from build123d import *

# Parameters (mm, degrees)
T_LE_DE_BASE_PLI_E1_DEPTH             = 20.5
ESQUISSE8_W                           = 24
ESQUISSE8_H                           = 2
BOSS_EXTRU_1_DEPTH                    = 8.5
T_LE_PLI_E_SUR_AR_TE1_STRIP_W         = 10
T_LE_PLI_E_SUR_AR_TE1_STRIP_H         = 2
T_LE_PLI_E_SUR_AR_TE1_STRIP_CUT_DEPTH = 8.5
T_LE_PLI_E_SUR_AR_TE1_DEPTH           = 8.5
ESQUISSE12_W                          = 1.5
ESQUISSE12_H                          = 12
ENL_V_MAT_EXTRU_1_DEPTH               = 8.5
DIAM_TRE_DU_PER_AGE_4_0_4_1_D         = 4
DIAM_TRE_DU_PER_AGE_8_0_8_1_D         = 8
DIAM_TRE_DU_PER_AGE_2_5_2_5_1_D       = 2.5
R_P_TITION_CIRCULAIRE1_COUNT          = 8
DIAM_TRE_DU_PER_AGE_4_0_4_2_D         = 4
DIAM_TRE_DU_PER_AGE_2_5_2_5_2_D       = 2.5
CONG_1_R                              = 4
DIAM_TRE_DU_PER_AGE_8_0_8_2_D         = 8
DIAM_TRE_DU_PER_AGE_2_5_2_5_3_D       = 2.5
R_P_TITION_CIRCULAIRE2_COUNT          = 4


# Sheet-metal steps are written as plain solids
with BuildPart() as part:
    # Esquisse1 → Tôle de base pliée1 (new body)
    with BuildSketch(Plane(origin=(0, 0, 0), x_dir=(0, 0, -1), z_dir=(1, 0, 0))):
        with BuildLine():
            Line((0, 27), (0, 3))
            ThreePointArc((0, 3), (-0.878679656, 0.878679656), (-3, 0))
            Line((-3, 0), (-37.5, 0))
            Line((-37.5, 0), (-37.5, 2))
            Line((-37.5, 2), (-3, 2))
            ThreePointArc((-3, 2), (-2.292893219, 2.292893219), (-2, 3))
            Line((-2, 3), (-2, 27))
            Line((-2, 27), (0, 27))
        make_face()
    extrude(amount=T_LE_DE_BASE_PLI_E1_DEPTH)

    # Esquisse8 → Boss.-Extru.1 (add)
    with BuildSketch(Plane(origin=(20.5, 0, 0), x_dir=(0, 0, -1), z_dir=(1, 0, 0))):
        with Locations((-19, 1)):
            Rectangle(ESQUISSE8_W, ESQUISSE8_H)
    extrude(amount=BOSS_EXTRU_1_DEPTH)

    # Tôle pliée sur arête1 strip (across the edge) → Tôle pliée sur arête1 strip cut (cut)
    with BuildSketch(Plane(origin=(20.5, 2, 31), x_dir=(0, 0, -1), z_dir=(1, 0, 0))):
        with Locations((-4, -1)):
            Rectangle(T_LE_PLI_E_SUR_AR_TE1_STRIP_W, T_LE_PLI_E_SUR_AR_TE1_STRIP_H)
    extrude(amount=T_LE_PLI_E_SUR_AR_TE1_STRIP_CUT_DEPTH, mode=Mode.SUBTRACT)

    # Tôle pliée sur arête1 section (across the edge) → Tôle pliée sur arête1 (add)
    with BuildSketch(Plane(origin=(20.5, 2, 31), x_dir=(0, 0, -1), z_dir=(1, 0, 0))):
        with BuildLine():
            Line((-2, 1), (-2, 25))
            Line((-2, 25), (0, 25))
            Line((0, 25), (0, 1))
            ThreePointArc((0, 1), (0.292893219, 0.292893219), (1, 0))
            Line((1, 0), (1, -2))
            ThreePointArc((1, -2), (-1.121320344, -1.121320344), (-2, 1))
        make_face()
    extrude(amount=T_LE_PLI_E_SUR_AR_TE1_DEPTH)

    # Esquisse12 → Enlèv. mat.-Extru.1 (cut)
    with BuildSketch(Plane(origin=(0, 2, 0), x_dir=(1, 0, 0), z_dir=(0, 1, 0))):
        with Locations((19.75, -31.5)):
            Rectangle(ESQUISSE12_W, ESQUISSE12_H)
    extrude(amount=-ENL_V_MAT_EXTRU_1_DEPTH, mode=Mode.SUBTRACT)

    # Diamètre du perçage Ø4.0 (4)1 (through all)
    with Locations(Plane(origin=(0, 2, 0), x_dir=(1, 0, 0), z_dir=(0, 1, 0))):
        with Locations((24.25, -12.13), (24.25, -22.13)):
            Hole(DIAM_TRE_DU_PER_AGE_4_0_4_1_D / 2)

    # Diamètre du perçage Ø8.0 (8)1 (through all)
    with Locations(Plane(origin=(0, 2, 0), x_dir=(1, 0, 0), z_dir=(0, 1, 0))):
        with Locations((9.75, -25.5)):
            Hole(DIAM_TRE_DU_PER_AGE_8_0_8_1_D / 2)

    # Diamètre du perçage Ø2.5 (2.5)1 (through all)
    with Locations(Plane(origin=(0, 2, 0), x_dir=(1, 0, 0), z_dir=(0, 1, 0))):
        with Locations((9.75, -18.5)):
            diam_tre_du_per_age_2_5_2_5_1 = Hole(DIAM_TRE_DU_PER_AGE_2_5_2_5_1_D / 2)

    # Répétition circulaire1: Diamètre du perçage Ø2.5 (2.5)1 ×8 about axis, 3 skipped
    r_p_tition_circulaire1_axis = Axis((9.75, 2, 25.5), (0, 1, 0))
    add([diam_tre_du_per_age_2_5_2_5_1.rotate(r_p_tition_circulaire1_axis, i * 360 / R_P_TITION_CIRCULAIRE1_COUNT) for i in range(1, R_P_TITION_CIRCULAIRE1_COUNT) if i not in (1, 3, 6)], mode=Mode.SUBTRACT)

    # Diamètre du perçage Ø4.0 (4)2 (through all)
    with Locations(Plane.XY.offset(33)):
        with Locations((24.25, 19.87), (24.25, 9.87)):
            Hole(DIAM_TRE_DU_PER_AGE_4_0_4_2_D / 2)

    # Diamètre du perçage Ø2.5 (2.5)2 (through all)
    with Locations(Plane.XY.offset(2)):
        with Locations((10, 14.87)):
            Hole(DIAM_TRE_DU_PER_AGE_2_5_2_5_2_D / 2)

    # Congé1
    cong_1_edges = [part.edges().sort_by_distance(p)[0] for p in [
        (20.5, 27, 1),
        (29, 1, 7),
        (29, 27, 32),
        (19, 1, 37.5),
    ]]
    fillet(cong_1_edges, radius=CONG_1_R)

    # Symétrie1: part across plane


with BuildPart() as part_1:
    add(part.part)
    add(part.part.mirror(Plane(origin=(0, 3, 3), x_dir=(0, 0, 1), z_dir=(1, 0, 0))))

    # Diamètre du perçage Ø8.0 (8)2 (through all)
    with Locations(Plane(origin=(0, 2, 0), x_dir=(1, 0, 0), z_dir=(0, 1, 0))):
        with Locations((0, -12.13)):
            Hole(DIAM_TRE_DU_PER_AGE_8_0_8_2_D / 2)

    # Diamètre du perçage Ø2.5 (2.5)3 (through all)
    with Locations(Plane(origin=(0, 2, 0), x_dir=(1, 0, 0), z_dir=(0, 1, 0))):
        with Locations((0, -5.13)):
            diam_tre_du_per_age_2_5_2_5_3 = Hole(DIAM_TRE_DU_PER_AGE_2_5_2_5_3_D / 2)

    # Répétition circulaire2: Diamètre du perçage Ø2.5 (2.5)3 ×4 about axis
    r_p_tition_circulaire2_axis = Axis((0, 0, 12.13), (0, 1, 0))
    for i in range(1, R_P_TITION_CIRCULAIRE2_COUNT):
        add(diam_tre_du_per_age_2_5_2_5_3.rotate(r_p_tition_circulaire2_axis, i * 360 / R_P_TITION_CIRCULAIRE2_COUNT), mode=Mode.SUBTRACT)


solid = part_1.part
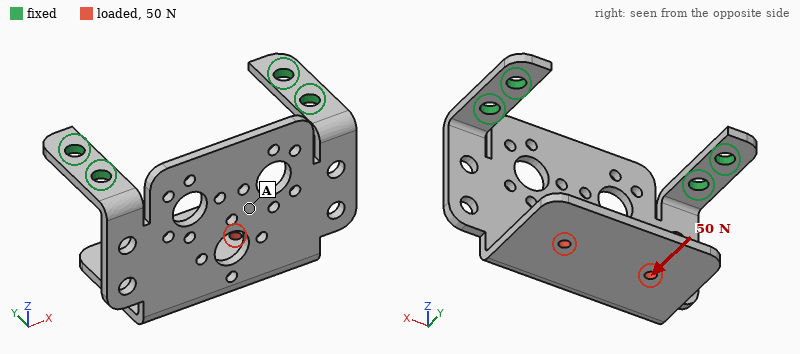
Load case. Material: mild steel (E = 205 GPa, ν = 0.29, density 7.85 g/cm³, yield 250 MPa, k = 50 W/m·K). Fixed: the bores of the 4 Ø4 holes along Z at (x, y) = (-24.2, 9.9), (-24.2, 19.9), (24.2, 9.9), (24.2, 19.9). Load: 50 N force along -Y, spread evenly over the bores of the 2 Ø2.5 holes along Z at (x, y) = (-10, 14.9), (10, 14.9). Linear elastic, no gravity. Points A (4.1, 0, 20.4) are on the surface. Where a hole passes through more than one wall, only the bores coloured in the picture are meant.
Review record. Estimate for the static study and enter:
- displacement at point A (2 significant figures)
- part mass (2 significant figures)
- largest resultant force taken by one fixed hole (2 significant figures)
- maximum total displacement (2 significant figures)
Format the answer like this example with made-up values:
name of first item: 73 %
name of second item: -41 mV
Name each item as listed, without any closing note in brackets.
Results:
displacement at point A: 0.10 mm
part mass: 47 g
largest resultant force taken by one fixed hole: 24 N
maximum total displacement: 0.47 mm
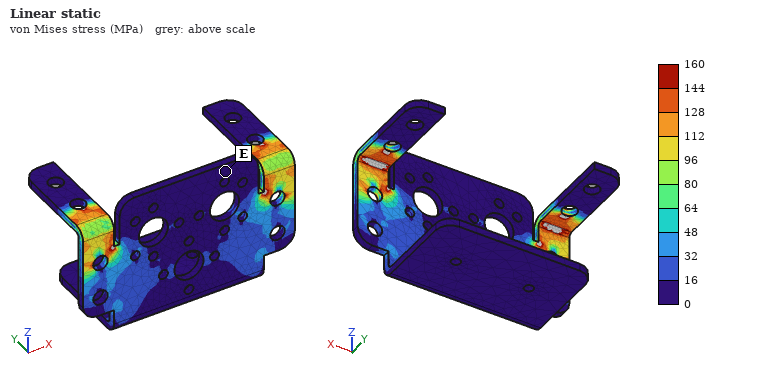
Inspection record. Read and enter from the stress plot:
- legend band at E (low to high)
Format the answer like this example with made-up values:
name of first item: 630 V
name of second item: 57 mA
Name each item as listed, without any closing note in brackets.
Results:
legend band at E: 0 to 16 MPa
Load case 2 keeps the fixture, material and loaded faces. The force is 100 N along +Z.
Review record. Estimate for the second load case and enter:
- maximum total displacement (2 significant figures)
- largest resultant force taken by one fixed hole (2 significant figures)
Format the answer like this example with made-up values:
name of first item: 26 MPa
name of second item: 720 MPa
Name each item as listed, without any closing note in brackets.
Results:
maximum total displacement: 0.53 mm
largest resultant force taken by one fixed hole: 52 N
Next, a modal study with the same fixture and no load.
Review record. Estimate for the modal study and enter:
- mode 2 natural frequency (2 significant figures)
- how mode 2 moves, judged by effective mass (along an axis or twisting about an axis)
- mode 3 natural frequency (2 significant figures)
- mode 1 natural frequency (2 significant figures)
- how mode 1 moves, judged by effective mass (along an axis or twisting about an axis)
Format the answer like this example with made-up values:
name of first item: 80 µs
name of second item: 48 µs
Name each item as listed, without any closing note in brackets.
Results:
mode 2 natural frequency: 1100 Hz
how mode 2 moves, judged by effective mass: along X
mode 3 natural frequency: 1400 Hz
mode 1 natural frequency: 370 Hz
how mode 1 moves, judged by effective mass: along Y
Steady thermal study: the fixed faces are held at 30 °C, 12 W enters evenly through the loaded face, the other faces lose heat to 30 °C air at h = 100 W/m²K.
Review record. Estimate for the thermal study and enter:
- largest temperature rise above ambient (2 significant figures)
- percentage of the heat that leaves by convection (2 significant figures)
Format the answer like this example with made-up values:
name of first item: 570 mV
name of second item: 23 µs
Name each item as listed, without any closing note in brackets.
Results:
largest temperature rise above ambient: 52 K
percentage of the heat that leaves by convection: 96 %
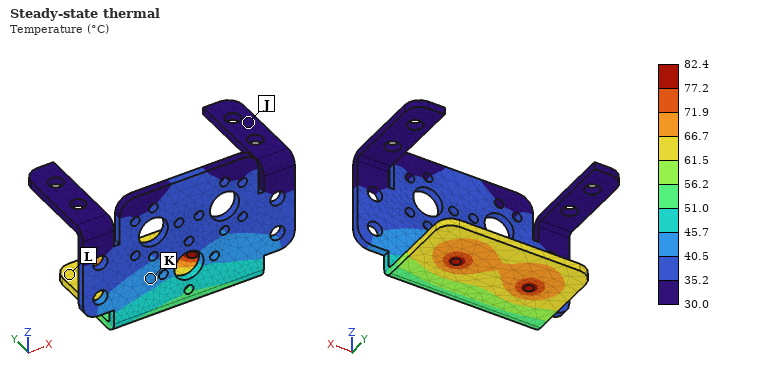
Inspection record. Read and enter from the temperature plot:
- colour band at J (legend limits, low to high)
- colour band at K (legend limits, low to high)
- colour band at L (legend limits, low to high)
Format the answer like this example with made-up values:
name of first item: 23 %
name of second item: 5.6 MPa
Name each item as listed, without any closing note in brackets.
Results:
colour band at J: 30.0 to 35.2 °C
colour band at K: 40.5 to 45.7 °C
colour band at L: 61.5 to 66.7 °C
